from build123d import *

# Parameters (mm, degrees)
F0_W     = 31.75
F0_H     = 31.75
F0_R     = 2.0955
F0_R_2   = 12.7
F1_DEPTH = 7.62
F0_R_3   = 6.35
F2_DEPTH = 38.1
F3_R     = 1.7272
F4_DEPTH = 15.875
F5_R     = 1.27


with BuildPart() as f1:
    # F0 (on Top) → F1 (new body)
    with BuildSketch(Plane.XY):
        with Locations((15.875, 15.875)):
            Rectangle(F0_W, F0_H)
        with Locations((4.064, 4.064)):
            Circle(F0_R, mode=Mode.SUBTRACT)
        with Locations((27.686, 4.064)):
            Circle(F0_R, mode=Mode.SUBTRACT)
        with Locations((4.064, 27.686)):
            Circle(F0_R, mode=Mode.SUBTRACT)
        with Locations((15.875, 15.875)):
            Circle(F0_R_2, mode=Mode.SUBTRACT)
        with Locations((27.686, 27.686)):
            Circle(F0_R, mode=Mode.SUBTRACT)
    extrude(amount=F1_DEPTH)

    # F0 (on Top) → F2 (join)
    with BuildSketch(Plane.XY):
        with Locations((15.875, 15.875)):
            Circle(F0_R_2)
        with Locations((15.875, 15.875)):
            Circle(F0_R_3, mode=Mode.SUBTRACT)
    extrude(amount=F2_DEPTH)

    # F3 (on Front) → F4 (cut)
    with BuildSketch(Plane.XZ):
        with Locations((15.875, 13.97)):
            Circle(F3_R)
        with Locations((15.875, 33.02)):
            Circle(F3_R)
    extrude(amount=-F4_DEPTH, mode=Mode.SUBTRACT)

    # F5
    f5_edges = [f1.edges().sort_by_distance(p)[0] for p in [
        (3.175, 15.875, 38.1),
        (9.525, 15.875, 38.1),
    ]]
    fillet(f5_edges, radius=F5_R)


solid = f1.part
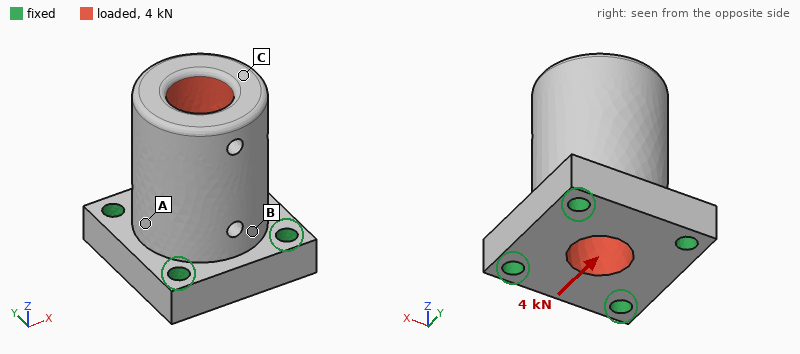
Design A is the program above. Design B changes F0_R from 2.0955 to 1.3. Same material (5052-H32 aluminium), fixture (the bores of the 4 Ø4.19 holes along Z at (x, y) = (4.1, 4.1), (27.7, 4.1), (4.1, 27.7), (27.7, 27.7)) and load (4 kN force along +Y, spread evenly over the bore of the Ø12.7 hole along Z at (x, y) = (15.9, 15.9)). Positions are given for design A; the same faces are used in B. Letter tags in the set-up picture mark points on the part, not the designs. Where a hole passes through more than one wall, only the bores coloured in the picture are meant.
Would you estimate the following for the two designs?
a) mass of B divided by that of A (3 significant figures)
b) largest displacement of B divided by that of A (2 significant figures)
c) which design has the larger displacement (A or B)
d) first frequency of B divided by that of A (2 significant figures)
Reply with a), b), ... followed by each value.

a) 1.01
b) 1.1
c) B
d) 0.94
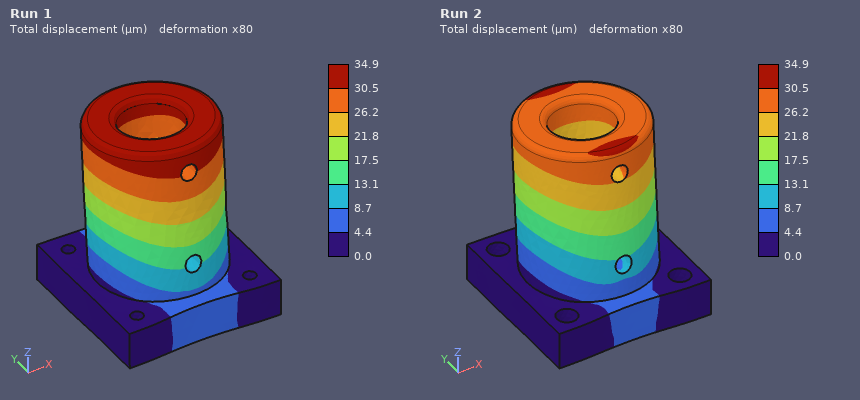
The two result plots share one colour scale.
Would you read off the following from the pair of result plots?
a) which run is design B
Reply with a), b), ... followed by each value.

a) Run 1
